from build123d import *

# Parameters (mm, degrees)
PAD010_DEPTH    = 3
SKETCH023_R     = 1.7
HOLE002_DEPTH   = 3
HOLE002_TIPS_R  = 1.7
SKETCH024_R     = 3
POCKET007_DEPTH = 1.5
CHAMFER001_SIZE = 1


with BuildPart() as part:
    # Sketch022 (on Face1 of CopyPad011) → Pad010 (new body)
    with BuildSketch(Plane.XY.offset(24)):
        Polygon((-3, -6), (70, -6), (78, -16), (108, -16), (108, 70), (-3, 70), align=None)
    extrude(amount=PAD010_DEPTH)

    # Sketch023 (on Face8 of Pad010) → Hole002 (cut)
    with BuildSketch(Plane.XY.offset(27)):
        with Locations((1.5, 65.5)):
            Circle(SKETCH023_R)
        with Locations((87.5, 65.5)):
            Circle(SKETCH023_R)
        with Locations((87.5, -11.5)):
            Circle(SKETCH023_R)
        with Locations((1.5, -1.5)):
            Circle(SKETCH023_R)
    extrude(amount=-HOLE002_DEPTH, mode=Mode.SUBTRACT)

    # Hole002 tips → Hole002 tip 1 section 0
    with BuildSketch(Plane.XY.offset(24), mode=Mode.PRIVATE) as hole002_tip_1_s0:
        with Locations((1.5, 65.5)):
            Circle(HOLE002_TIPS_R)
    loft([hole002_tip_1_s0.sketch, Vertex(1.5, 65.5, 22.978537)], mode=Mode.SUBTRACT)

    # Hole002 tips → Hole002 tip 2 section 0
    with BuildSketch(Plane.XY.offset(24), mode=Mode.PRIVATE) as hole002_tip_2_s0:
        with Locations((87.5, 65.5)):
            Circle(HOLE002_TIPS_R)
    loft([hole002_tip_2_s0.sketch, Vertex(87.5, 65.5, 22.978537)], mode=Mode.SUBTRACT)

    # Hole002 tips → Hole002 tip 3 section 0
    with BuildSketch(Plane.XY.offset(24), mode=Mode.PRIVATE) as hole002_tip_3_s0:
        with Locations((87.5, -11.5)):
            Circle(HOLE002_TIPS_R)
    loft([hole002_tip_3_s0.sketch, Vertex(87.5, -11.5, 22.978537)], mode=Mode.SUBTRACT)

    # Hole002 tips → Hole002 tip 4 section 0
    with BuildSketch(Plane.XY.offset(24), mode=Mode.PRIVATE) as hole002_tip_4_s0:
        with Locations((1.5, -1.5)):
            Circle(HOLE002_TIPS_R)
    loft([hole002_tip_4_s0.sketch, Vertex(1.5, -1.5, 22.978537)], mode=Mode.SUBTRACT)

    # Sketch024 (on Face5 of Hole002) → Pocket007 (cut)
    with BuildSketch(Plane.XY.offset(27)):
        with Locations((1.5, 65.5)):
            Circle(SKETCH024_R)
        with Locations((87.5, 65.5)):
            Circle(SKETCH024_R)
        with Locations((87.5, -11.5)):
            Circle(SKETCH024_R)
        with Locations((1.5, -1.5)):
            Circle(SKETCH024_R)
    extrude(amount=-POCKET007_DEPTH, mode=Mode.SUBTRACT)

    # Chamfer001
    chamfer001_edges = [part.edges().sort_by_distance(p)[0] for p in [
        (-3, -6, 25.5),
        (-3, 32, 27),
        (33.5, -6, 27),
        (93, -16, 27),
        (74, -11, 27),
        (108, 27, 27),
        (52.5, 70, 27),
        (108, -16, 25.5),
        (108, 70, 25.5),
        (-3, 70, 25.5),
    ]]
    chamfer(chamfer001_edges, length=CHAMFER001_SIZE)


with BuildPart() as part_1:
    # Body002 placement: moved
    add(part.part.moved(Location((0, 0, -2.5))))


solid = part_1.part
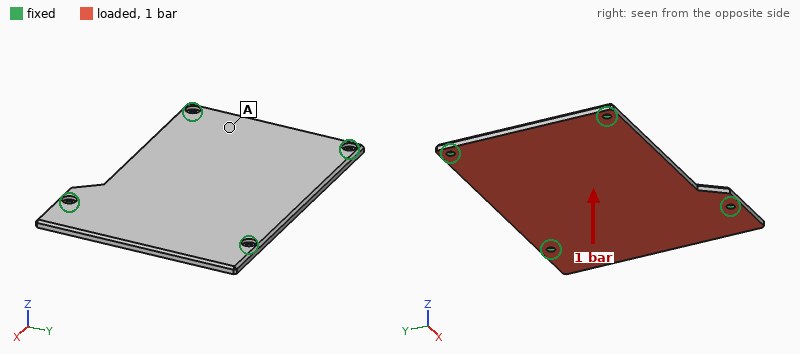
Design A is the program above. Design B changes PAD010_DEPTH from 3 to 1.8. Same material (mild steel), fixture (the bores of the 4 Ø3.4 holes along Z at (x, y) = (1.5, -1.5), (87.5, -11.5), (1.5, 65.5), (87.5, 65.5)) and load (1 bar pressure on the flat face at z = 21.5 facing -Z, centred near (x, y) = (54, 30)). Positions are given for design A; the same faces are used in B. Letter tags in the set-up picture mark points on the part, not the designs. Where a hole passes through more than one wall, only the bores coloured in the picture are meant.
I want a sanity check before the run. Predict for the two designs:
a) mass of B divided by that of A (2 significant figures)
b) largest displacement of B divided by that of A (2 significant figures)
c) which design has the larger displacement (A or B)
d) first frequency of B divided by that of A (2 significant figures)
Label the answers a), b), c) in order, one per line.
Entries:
a) 0.60
b) 3.7
c) B
d) 0.68
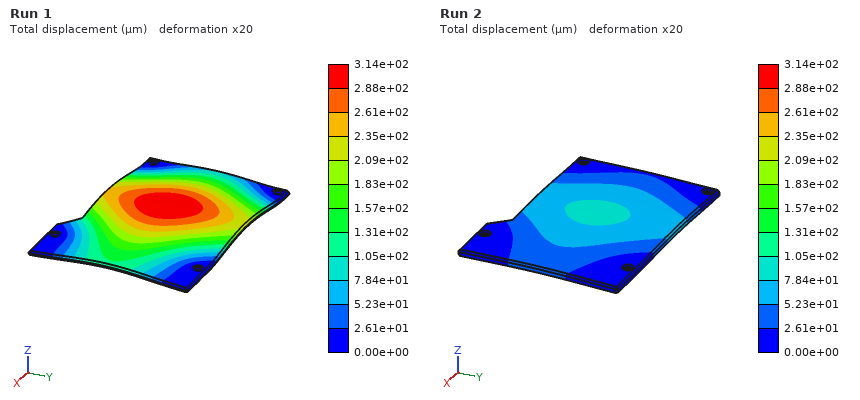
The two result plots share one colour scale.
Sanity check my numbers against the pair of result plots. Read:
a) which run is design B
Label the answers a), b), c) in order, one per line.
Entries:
a) Run 1
